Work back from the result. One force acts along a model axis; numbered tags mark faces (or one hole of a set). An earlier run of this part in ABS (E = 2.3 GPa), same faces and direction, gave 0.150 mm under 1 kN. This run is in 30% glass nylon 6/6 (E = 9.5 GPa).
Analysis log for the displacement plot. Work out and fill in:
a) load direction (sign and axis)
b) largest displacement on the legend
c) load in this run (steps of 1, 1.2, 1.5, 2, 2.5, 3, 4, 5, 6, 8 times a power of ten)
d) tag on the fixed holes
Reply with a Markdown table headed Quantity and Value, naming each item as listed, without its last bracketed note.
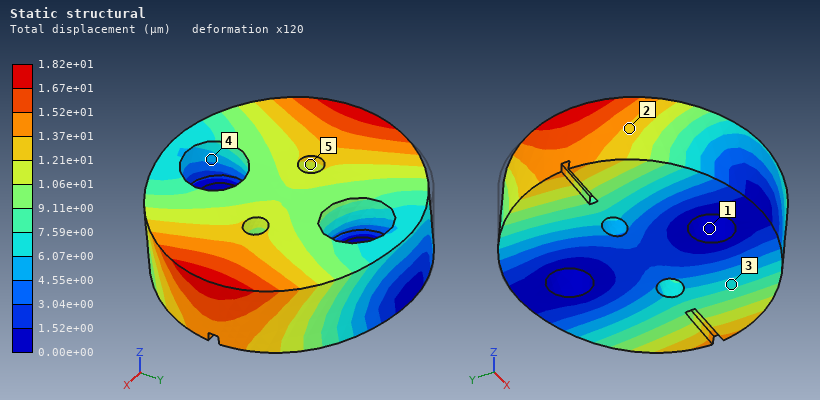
| Quantity | Value |
|---|---|
| load direction | +X |
| largest displacement on the legend | 1.82e+01 µm |
| load in this run | 500 N |
| tag on the fixed holes | 1 |
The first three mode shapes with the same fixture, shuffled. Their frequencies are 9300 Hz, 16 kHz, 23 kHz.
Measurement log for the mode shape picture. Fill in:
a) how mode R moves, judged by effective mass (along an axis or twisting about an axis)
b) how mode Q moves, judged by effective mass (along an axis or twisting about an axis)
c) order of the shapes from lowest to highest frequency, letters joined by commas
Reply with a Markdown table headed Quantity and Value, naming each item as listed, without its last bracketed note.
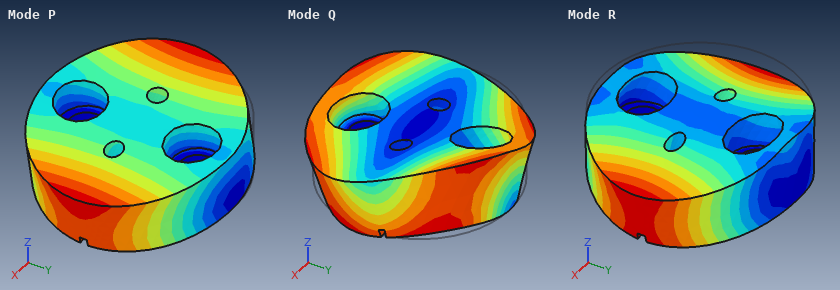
| Quantity | Value |
|---|---|
| how mode R moves, judged by effective mass | along Z |
| how mode Q moves, judged by effective mass | twisting about Z |
| order of the shapes from lowest to highest frequency, letters joined by commas | P, R, Q |
